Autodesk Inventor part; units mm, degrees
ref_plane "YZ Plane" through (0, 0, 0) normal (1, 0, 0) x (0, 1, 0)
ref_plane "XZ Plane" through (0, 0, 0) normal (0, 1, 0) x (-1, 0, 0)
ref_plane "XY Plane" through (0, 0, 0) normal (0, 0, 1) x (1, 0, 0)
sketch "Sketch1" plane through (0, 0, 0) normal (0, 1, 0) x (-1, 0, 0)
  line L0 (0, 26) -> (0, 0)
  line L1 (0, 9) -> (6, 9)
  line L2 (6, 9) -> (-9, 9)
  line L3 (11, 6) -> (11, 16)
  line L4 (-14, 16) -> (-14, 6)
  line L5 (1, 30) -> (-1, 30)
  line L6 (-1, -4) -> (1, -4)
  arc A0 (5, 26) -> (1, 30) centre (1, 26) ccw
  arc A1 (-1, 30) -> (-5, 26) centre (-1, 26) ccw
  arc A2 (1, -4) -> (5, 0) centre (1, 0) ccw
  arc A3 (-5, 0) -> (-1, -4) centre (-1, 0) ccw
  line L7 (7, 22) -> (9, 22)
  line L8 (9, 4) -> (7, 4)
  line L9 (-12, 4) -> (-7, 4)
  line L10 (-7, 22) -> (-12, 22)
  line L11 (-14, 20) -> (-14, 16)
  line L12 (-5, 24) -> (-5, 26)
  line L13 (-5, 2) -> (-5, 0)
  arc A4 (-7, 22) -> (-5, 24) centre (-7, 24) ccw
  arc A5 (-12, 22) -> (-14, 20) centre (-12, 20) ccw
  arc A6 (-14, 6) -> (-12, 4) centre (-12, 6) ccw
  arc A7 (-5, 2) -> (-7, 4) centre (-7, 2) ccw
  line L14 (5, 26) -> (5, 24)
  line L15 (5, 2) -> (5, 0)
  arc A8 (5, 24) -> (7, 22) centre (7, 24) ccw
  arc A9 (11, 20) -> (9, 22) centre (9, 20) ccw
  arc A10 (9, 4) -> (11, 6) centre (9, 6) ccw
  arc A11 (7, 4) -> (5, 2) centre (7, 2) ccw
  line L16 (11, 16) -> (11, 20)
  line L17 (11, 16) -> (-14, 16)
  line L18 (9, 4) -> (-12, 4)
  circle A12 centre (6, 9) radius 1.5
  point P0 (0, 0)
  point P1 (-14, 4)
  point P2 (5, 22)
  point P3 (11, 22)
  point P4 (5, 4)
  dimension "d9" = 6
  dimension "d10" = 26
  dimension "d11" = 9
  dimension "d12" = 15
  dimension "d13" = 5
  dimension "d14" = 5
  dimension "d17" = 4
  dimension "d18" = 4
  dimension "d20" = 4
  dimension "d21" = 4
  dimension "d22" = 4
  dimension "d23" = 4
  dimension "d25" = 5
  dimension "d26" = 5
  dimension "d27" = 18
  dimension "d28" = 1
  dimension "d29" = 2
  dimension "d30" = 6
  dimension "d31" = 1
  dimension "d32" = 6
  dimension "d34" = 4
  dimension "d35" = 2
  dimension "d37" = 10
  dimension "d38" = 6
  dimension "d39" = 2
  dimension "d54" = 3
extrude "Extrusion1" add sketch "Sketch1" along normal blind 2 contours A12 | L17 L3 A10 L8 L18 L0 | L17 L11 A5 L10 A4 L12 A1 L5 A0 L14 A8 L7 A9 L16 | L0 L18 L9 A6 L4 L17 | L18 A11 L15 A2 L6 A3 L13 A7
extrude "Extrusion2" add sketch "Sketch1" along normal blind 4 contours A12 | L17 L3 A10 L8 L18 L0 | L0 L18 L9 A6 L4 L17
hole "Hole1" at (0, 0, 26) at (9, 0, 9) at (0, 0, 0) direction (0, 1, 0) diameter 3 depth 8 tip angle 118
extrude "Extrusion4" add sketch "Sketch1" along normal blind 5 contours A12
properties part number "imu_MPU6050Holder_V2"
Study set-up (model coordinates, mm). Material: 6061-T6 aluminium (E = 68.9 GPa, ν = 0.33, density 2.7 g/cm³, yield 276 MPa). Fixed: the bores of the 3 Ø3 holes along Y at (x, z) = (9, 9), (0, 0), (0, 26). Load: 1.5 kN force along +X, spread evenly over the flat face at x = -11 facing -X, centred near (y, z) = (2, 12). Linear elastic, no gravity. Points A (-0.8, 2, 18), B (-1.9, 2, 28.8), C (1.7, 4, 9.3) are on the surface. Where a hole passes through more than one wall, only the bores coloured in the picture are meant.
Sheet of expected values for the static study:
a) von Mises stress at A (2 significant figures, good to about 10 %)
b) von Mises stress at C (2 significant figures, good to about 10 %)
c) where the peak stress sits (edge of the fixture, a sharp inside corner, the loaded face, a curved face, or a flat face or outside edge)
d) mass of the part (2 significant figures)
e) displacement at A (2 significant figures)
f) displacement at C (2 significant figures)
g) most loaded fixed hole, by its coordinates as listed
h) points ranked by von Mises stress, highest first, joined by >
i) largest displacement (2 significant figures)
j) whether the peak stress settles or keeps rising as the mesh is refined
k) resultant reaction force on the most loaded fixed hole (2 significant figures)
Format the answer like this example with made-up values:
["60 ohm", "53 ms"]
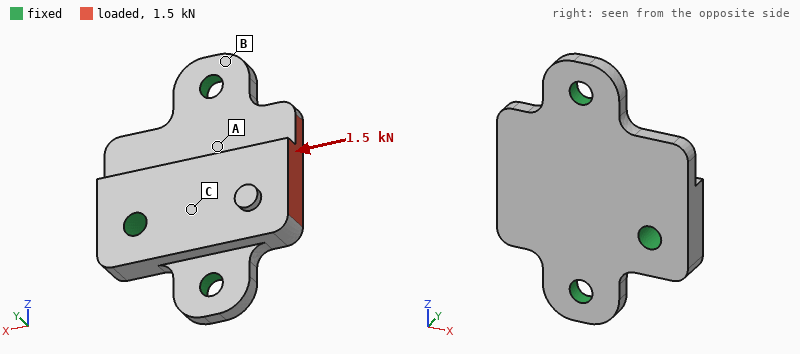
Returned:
["17 MPa", "32 MPa", "edge of the fixture", "4.7 g", "4.2 µm", "3.3 µm", "(9, 9)", "C > A > B", "11 µm", "keeps rising", "980 N"]
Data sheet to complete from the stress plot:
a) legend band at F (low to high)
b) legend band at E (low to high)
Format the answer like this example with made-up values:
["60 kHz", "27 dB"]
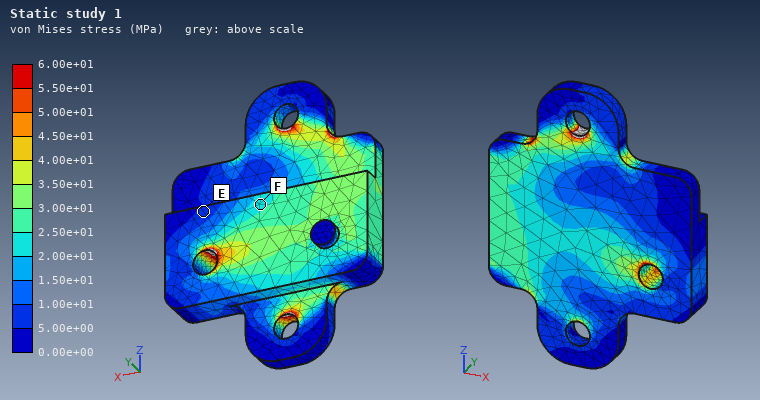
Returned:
["2.00e+01 to 2.50e+01 MPa", "5.00e+00 to 1.00e+01 MPa"]
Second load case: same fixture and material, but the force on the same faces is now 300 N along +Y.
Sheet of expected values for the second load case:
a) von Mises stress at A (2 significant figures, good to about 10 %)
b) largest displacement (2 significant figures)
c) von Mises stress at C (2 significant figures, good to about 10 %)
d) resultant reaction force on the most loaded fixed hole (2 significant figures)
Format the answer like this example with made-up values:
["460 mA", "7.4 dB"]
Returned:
["44 MPa", "84 µm", "66 MPa", "350 N"]
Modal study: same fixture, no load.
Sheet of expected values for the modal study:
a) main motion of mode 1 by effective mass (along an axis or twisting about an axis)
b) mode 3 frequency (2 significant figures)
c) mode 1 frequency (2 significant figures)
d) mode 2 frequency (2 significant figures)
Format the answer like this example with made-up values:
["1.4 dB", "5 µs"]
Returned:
["along Y", "32 kHz", "12 kHz", "30 kHz"]
